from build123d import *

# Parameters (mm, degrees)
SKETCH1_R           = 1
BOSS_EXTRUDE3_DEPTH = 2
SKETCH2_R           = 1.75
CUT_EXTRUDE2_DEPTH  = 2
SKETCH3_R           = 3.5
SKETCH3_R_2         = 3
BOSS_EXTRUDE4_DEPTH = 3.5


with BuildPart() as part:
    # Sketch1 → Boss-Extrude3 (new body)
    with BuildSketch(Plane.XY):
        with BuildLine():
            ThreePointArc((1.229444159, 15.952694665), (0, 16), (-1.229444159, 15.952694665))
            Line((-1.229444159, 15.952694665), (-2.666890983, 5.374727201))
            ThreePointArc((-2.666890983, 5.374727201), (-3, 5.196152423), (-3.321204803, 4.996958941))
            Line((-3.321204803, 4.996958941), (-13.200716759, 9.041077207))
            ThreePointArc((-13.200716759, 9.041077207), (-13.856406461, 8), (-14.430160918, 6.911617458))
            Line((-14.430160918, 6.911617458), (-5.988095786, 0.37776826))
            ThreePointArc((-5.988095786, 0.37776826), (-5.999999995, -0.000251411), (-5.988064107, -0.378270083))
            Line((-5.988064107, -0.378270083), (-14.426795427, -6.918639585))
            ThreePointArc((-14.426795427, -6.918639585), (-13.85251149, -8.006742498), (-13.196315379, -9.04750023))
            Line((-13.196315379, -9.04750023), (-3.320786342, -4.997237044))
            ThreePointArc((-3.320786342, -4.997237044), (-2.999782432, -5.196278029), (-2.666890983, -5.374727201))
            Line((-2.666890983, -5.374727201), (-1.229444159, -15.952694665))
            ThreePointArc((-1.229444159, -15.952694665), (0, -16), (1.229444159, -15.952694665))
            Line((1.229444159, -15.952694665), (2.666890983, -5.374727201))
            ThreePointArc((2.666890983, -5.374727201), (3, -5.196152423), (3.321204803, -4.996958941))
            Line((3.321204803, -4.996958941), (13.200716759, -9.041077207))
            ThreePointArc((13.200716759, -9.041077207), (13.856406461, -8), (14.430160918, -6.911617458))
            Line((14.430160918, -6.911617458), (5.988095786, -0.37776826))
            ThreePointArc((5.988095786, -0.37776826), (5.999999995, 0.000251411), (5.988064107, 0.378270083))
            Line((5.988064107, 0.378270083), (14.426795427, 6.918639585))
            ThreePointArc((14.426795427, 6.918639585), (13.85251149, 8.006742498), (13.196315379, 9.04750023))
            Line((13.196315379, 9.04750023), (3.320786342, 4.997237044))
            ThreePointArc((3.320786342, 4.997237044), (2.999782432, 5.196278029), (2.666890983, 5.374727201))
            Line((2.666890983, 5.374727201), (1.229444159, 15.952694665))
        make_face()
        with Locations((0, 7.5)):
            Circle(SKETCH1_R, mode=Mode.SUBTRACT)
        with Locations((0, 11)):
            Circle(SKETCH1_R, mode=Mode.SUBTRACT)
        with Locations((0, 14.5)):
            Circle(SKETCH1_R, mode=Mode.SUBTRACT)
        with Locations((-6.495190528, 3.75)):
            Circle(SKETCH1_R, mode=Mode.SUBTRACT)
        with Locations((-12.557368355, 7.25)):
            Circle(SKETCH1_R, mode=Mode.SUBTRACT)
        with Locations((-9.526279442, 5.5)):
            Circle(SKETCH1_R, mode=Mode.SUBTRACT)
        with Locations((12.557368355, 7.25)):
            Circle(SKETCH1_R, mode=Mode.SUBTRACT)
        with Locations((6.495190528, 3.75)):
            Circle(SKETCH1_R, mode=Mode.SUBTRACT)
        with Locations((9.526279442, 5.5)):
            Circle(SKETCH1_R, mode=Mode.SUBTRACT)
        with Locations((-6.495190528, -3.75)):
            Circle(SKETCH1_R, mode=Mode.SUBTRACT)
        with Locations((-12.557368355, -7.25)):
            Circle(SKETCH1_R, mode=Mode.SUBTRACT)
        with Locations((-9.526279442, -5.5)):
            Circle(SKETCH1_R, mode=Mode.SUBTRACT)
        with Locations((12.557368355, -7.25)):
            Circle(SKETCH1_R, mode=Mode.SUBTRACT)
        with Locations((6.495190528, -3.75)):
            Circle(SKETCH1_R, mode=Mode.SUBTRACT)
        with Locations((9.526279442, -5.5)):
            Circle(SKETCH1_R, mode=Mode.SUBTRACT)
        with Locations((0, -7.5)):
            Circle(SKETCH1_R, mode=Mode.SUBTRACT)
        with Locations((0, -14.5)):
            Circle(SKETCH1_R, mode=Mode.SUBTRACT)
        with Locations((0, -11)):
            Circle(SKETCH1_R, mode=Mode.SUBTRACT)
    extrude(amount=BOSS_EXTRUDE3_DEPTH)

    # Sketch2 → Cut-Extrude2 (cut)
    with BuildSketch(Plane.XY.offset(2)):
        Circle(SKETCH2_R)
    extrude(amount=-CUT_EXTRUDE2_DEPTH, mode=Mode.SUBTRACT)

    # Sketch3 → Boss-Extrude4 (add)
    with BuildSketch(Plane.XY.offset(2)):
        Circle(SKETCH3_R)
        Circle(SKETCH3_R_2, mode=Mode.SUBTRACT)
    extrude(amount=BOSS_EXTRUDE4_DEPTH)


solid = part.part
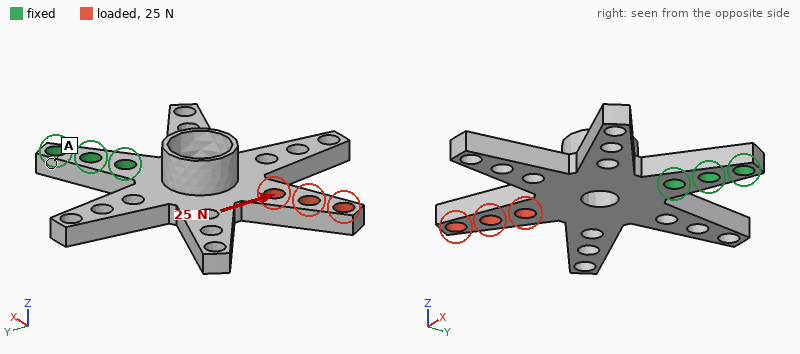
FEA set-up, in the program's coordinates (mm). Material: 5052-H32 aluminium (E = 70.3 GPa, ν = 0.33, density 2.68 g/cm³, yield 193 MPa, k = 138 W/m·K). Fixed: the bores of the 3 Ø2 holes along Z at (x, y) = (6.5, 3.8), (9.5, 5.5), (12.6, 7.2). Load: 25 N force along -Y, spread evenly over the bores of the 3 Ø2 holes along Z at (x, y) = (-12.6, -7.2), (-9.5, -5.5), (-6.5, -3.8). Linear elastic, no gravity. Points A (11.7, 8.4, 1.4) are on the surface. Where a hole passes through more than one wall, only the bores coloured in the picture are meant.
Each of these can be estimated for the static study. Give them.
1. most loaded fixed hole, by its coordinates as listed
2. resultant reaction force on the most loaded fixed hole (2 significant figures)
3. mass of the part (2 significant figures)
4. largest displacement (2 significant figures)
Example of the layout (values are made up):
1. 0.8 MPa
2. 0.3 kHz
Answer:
1. (6.5, 3.8)
2. 55 N
3. 1.6 g
4. 34 µm
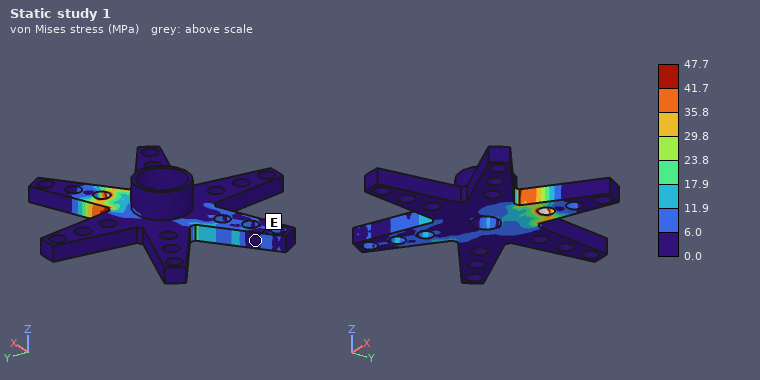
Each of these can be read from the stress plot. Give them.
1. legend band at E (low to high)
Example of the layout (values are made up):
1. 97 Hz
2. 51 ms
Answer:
1. 0.0 to 6.0 MPa
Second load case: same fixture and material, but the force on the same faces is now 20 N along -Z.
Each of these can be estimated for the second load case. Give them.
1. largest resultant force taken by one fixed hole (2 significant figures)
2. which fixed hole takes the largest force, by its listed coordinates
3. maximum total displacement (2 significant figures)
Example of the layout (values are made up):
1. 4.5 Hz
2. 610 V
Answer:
1. 30 N
2. (6.5, 3.8)
3. 0.18 mm
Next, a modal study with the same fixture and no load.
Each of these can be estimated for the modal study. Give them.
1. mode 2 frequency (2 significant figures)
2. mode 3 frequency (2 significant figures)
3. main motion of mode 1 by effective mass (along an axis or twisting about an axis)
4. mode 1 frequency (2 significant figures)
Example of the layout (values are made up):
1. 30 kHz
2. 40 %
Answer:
1. 5500 Hz
2. 6400 Hz
3. along Z
4. 3700 Hz
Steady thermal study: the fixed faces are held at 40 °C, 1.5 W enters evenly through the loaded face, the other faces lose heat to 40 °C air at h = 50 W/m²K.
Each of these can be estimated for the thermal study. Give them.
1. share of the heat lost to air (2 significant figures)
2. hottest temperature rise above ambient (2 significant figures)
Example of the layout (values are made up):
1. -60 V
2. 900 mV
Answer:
1. 19 %
2. 19 K
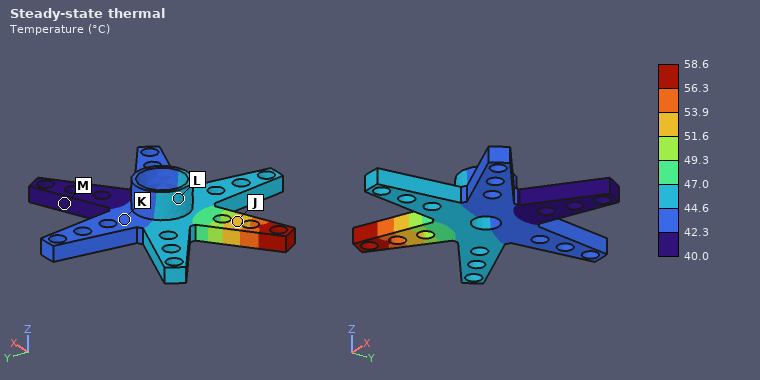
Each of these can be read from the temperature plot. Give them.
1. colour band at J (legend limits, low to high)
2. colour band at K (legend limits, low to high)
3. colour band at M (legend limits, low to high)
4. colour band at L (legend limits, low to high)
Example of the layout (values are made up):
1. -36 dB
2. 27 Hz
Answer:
1. 51.6 to 53.9 °C
2. 42.3 to 44.6 °C
3. 40.0 to 42.3 °C
4. 44.6 to 47.0 °C
